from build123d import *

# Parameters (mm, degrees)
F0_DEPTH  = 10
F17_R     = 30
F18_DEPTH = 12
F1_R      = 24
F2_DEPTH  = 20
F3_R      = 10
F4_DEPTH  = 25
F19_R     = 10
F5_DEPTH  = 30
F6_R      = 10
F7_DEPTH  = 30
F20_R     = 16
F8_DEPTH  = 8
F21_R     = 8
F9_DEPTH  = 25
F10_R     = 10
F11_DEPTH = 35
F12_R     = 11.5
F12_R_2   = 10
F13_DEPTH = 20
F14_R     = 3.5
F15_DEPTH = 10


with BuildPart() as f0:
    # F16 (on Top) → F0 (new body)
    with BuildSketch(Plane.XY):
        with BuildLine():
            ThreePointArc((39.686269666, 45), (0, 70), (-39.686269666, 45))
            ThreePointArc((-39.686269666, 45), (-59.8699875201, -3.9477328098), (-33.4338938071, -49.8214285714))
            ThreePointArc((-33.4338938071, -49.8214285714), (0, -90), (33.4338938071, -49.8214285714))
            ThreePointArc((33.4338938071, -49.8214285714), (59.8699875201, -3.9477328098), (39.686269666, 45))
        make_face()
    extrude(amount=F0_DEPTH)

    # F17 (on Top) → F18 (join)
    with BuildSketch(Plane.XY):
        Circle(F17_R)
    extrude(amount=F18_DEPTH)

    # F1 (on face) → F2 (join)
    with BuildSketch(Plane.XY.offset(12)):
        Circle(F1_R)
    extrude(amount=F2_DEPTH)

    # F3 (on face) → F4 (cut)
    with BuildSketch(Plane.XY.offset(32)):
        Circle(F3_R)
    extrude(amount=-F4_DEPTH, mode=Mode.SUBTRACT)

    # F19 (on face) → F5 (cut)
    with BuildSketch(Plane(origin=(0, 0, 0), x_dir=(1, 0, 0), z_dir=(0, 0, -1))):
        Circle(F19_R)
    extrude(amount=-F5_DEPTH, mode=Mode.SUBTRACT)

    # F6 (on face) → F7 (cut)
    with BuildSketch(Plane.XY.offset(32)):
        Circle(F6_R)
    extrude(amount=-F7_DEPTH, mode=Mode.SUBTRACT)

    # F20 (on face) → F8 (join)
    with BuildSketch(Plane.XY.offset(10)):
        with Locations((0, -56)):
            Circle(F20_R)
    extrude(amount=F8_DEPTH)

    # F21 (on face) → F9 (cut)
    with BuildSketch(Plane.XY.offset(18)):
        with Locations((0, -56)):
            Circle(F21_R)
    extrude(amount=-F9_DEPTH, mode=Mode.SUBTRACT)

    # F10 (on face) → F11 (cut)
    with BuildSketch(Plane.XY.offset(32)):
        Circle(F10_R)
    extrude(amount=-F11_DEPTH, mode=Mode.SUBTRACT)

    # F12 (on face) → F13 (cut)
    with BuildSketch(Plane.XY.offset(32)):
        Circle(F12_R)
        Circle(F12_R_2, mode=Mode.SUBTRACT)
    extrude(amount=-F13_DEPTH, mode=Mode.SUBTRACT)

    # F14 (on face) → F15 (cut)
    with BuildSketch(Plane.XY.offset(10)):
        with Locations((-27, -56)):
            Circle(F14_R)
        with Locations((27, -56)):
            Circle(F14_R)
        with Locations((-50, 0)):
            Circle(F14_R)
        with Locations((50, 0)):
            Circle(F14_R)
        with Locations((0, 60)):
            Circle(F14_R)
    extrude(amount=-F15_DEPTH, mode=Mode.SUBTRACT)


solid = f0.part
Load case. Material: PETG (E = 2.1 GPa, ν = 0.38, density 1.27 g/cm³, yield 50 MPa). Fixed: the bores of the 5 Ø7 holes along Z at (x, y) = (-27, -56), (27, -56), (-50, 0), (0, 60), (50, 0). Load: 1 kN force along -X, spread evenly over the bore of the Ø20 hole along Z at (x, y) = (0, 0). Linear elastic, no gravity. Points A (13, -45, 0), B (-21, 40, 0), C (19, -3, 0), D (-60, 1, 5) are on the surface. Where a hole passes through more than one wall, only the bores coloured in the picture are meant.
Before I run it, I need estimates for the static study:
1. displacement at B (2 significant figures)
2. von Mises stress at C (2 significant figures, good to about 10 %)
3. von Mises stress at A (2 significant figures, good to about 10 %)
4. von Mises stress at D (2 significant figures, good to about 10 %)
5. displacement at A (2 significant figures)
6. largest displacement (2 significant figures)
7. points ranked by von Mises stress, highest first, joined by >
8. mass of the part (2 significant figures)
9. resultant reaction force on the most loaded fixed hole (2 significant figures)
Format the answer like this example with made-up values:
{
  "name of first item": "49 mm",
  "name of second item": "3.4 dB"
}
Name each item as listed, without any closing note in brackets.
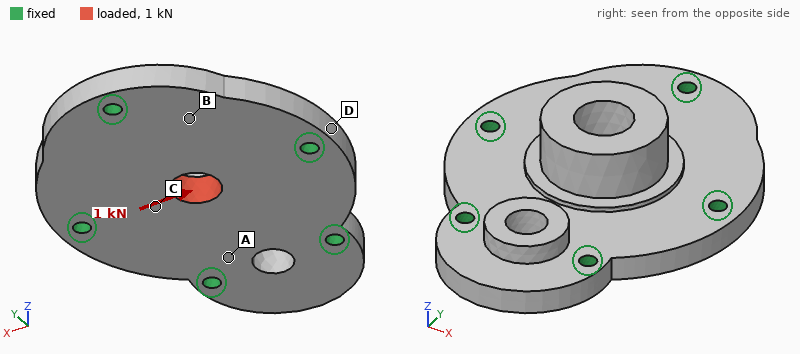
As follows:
{
  "displacement at B": "12 µm",
  "von Mises stress at C": "1.4 MPa",
  "von Mises stress at A": "0.46 MPa",
  "von Mises stress at D": "0.92 MPa",
  "displacement at A": "5.0 µm",
  "largest displacement": "28 µm",
  "points ranked by von Mises stress, highest first, joined by >": "C > D > A > B",
  "mass of the part": "210 g",
  "resultant reaction force on the most loaded fixed hole": "340 N"
}
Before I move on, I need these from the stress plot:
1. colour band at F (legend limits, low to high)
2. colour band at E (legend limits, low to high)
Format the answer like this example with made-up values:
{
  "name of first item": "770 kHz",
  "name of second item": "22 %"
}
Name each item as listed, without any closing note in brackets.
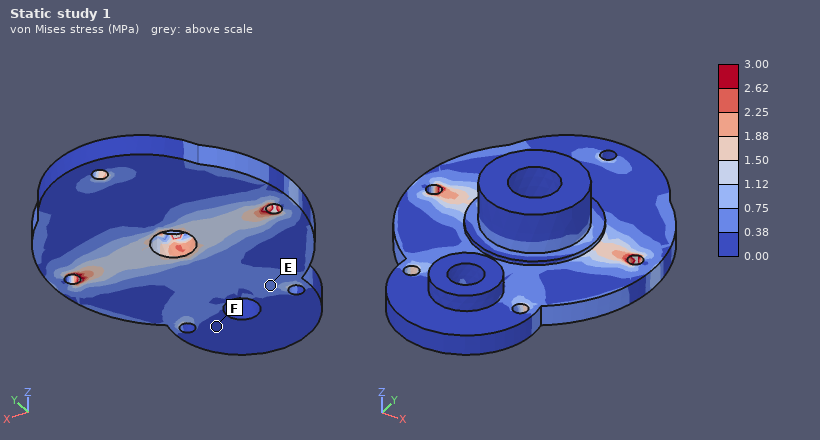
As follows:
{
  "colour band at F": "0.00 to 0.38 MPa",
  "colour band at E": "0.38 to 0.75 MPa"
}
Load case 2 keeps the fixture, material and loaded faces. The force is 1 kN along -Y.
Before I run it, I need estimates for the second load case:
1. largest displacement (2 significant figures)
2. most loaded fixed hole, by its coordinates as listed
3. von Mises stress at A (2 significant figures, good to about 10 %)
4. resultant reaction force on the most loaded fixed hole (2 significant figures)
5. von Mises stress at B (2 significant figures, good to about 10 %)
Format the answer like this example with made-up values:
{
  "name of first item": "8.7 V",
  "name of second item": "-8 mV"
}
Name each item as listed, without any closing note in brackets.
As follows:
{
  "largest displacement": "28 µm",
  "most loaded fixed hole, by its coordinates as listed": "(0, 60)",
  "von Mises stress at A": "0.84 MPa",
  "resultant reaction force on the most loaded fixed hole": "260 N",
  "von Mises stress at B": "0.36 MPa"
}
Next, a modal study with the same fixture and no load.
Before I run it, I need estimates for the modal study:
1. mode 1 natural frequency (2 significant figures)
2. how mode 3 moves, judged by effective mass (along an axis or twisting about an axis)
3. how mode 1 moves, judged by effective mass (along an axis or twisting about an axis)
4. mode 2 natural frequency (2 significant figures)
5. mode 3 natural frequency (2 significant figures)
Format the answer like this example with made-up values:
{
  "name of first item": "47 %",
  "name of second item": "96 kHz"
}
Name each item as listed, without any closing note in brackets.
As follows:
{
  "mode 1 natural frequency": "1400 Hz",
  "how mode 3 moves, judged by effective mass": "twisting about Y",
  "how mode 1 moves, judged by effective mass": "along Z",
  "mode 2 natural frequency": "1800 Hz",
  "mode 3 natural frequency": "1900 Hz"
}
